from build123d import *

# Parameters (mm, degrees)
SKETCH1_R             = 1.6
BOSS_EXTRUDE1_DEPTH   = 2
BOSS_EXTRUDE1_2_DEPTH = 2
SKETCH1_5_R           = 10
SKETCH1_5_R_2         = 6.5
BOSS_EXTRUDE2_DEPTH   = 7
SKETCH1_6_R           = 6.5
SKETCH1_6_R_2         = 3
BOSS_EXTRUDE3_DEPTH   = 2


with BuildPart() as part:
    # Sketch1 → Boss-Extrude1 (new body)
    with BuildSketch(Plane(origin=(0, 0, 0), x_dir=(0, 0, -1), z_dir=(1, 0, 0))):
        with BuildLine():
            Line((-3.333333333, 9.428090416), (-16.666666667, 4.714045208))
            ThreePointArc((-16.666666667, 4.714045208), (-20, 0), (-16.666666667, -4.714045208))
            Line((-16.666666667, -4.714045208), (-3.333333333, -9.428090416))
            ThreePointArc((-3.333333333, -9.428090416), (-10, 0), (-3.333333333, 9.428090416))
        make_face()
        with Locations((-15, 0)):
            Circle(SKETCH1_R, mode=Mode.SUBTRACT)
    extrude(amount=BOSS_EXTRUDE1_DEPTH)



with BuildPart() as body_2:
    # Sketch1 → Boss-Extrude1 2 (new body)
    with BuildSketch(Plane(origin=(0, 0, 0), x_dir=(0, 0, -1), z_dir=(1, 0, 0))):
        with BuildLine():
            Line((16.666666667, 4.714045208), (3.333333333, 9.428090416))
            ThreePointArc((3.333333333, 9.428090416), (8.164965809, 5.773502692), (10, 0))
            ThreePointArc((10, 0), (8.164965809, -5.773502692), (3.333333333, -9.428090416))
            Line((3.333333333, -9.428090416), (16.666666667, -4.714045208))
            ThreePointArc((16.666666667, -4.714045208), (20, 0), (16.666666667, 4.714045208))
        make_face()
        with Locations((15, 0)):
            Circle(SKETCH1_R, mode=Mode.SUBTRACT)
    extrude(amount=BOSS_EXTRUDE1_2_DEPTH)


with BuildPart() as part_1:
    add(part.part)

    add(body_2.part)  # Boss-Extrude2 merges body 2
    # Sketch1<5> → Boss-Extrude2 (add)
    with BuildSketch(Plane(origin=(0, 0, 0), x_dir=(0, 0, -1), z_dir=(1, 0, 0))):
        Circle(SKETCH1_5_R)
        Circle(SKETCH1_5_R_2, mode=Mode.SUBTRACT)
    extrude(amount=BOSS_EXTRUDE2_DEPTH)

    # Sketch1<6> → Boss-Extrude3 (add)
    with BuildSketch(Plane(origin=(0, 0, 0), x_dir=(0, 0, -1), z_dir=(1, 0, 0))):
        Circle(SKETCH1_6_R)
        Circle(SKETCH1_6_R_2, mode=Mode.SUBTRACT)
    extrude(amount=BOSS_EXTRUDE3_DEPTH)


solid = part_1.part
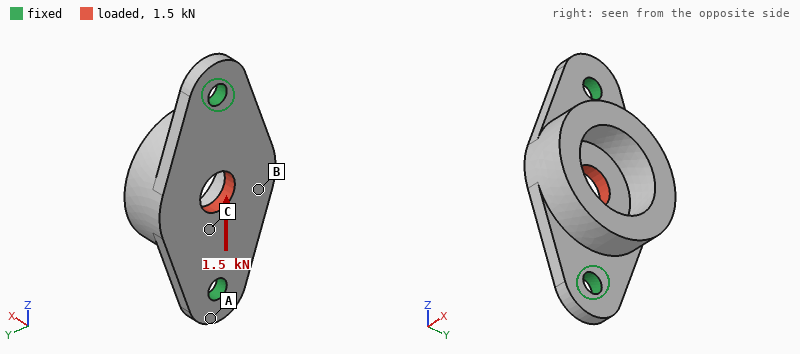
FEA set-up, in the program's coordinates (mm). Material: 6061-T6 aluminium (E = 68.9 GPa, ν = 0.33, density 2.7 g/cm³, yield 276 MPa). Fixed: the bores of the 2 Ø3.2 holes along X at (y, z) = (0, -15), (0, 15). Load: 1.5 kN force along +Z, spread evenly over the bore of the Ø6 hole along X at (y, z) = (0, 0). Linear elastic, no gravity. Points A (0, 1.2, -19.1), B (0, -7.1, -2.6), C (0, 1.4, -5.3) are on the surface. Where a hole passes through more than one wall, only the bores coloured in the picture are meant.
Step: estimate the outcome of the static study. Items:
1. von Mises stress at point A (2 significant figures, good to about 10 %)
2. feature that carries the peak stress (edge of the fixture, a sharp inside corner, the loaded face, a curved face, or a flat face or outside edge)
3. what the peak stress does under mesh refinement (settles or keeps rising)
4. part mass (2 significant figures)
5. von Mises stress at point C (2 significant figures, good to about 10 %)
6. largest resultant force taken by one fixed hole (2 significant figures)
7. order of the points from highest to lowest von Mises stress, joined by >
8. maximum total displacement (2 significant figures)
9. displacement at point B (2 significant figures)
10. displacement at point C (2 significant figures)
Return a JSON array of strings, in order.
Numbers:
["13 MPa", "edge of the fixture", "keeps rising", "5.2 g", "40 MPa", "750 N", "C > A > B", "7.3 µm", "4.8 µm", "5.4 µm"]
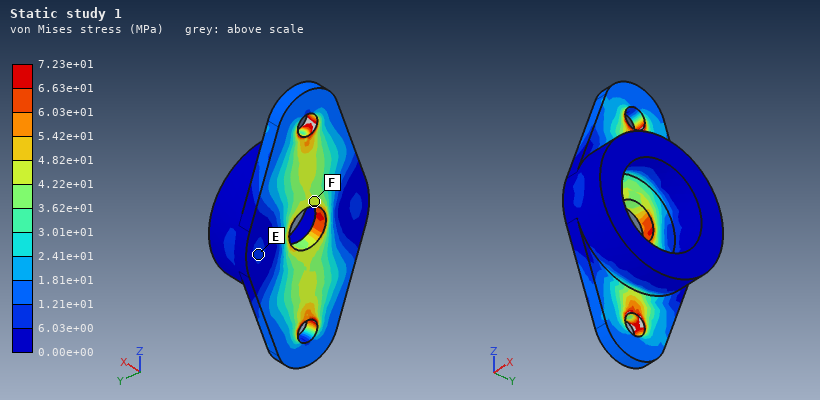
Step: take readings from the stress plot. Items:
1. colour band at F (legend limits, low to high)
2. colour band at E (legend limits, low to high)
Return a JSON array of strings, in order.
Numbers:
["4.22e+01 to 4.82e+01 MPa", "6.03e+00 to 1.21e+01 MPa"]
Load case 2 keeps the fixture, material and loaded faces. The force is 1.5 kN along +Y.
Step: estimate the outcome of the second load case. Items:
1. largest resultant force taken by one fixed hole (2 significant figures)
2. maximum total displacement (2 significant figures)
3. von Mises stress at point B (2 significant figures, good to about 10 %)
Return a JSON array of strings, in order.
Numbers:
["750 N", "18 µm", "41 MPa"]
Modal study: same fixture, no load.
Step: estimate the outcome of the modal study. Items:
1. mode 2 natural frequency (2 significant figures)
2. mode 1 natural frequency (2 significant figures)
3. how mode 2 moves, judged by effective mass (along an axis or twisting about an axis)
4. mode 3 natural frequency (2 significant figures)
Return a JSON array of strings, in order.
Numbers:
["13 kHz", "7700 Hz", "along X", "28 kHz"]
